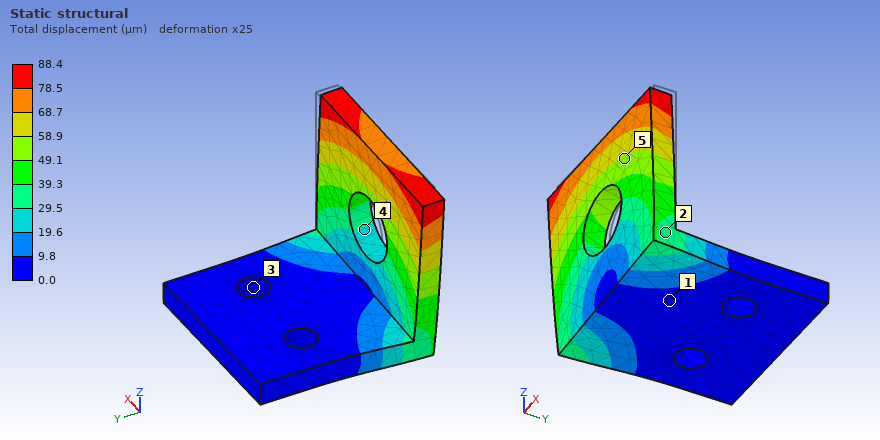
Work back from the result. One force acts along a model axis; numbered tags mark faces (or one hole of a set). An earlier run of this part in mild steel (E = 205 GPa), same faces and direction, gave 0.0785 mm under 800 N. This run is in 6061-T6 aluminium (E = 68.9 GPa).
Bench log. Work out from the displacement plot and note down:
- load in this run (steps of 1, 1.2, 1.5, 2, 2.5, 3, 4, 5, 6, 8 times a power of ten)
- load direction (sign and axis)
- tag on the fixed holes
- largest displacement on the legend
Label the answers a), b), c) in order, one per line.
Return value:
a) 300 N
b) -X
c) 3
d) 88.4 µm
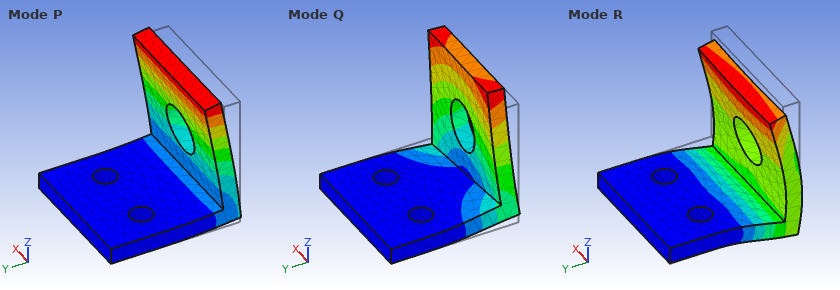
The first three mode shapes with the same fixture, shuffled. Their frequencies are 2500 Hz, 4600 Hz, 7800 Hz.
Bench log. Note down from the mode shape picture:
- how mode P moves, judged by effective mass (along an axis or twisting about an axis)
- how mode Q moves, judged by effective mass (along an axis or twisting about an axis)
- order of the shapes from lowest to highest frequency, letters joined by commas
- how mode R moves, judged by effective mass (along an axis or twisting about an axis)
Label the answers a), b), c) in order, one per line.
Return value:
a) along Y
b) along X
c) P, Q, R
d) along Z
